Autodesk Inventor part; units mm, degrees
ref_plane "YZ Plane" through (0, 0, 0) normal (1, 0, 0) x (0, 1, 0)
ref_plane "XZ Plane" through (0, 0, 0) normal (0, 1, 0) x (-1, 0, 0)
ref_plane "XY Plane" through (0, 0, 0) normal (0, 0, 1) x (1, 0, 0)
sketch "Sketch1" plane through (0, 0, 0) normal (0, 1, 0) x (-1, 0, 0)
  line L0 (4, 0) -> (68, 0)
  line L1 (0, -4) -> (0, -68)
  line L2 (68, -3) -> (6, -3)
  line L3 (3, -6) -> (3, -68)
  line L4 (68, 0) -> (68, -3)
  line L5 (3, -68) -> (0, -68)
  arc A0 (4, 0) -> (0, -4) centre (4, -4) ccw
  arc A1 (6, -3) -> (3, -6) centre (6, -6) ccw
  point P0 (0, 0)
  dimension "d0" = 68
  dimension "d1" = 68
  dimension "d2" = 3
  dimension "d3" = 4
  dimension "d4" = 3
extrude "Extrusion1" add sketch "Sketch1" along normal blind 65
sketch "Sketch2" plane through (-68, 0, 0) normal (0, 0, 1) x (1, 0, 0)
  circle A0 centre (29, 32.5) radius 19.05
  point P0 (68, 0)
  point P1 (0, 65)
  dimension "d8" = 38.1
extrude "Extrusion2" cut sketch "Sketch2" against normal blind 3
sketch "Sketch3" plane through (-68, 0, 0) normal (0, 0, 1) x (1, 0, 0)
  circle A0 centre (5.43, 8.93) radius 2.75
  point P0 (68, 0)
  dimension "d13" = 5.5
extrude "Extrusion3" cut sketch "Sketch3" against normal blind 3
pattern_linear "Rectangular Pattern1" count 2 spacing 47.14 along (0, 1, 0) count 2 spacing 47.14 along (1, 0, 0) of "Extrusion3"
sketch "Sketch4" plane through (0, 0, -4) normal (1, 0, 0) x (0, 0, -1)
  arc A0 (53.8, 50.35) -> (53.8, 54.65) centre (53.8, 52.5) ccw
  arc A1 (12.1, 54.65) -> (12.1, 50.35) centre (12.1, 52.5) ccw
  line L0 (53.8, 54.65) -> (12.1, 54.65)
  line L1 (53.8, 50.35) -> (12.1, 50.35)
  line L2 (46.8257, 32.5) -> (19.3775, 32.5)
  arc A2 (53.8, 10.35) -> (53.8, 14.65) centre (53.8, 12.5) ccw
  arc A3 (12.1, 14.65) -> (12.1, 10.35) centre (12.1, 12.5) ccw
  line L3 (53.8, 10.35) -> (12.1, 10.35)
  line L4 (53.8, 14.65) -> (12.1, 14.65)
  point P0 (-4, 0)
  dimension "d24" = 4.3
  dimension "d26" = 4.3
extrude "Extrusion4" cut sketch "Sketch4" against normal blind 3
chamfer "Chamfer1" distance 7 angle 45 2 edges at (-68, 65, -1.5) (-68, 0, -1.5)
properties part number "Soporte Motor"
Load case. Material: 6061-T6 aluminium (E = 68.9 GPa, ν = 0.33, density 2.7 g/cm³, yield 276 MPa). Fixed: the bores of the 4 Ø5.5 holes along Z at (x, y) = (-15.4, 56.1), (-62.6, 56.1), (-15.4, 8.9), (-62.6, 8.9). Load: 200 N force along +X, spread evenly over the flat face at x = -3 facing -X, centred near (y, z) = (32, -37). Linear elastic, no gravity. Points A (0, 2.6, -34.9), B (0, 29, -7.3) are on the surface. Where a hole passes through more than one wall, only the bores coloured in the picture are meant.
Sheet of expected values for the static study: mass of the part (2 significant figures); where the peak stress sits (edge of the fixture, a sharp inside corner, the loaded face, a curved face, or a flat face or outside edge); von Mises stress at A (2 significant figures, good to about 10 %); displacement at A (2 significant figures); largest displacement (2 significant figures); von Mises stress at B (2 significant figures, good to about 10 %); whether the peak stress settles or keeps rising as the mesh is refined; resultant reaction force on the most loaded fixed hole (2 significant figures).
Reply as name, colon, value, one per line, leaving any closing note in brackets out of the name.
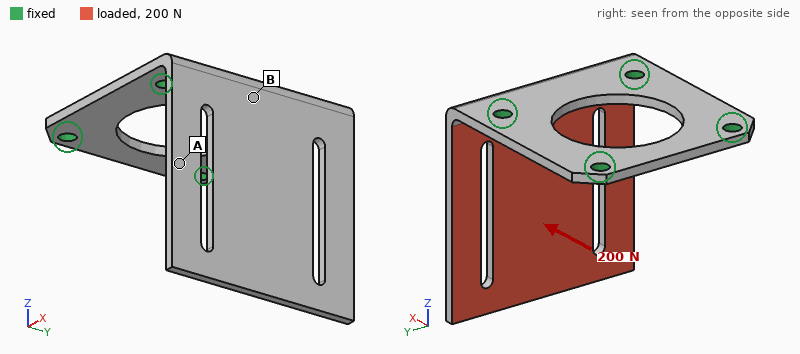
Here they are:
mass of the part: 56 g
where the peak stress sits: edge of the fixture
von Mises stress at A: 23 MPa
displacement at A: 0.53 mm
largest displacement: 1.3 mm
von Mises stress at B: 57 MPa
whether the peak stress settles or keeps rising as the mesh is refined: keeps rising
resultant reaction force on the most loaded fixed hole: 110 N
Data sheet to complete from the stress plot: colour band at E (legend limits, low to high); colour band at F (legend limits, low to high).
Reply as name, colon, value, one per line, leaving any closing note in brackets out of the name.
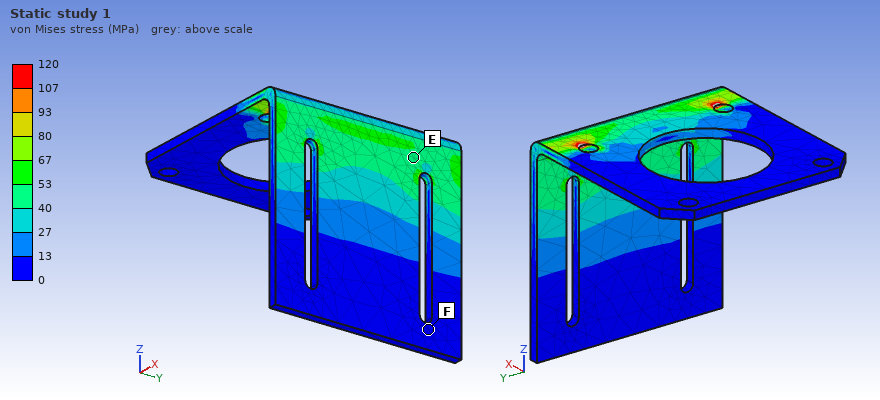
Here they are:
colour band at E: 40 to 53 MPa
colour band at F: 0 to 13 MPa
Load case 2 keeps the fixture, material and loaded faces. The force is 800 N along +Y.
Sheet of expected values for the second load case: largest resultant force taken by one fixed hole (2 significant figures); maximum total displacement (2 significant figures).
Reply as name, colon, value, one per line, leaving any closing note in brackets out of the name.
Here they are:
largest resultant force taken by one fixed hole: 730 N
maximum total displacement: 0.37 mm
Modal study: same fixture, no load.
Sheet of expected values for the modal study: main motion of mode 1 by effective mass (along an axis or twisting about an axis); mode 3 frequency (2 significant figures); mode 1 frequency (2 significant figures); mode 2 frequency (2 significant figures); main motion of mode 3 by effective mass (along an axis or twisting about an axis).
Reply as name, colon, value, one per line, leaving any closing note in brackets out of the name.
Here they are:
main motion of mode 1 by effective mass: along X
mode 3 frequency: 2100 Hz
mode 1 frequency: 450 Hz
mode 2 frequency: 1200 Hz
main motion of mode 3 by effective mass: along Y
